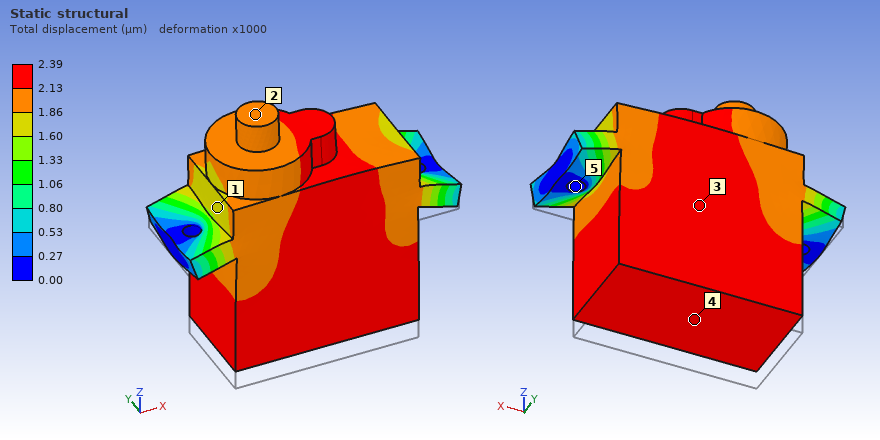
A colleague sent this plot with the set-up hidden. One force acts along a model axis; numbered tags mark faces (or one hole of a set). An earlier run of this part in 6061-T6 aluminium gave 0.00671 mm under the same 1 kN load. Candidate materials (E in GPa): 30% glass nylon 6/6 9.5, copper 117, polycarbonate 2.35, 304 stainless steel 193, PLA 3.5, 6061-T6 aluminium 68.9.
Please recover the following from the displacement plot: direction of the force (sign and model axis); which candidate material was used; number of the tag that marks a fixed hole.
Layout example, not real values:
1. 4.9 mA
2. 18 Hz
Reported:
1. +Z
2. 304 stainless steel
3. 5
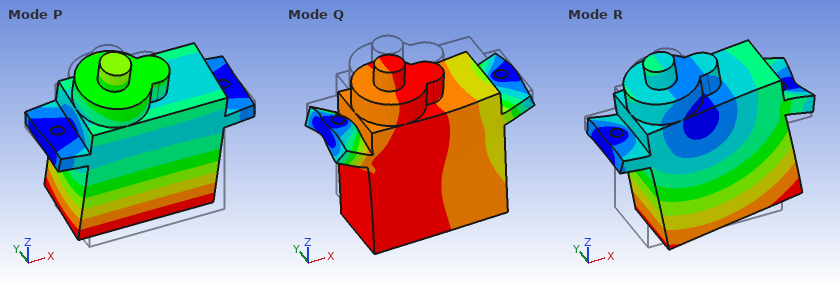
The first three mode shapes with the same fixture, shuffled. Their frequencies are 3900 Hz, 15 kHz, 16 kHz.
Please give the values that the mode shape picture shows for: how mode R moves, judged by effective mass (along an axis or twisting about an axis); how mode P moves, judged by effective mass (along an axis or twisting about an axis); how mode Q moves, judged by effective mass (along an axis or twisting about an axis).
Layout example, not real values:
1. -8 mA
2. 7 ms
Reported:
1. along X
2. along Y
3. along Z
